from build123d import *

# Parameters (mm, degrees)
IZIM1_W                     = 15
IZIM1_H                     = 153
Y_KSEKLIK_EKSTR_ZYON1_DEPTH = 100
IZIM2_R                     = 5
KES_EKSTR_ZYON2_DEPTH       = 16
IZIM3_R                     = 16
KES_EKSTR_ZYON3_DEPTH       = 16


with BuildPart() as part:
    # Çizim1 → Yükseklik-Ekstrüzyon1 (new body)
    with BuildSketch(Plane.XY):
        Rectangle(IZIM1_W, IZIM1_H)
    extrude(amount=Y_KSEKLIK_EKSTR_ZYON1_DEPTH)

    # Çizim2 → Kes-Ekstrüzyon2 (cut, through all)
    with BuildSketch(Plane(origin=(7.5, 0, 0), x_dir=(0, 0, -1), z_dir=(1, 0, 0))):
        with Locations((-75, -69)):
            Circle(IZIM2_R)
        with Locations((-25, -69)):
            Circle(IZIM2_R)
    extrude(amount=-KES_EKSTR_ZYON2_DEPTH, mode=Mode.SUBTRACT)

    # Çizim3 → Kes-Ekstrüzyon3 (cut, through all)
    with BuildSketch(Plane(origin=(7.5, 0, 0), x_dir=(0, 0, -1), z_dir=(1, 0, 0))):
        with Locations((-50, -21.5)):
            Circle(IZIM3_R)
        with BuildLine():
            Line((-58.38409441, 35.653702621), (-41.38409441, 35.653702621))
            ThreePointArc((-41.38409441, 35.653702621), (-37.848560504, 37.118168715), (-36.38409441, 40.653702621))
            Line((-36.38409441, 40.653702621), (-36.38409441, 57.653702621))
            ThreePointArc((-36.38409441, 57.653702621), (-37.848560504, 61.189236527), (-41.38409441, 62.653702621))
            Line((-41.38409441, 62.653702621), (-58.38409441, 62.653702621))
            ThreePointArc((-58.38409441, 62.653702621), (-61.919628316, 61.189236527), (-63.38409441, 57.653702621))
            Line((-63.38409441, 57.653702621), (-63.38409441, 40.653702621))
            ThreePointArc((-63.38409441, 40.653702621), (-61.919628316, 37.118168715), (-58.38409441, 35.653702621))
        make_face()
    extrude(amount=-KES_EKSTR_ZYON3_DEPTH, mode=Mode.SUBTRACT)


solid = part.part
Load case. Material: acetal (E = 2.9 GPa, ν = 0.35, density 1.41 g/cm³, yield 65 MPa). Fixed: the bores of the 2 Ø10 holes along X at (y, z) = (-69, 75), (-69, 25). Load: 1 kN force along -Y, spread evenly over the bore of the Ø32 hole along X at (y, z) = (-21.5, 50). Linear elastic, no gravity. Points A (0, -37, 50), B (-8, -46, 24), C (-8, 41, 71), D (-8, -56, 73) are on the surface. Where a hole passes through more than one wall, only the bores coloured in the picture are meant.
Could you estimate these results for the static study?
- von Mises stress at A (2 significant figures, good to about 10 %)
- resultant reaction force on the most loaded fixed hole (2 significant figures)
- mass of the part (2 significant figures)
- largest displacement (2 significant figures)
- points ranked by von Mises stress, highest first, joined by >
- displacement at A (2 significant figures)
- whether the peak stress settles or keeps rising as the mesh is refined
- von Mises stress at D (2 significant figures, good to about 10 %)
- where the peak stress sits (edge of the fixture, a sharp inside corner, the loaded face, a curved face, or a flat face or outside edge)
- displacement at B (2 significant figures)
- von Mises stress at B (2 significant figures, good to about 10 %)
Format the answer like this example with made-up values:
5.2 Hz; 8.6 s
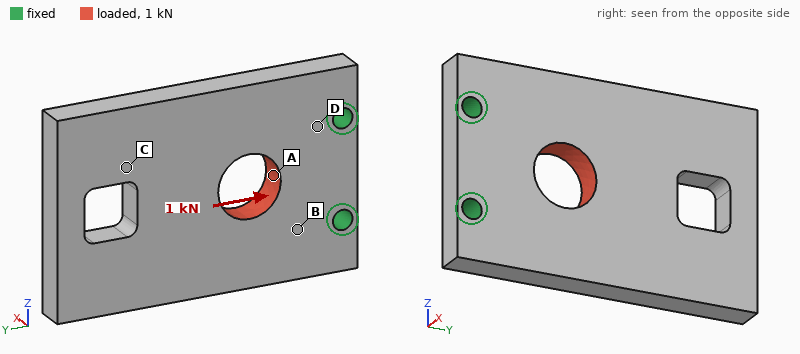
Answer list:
0.77 MPa; 500 N; 290 g; 25 µm; D > B > A > C; 11 µm; keeps rising; 1.4 MPa; edge of the fixture; 8.8 µm; 1.1 MPa
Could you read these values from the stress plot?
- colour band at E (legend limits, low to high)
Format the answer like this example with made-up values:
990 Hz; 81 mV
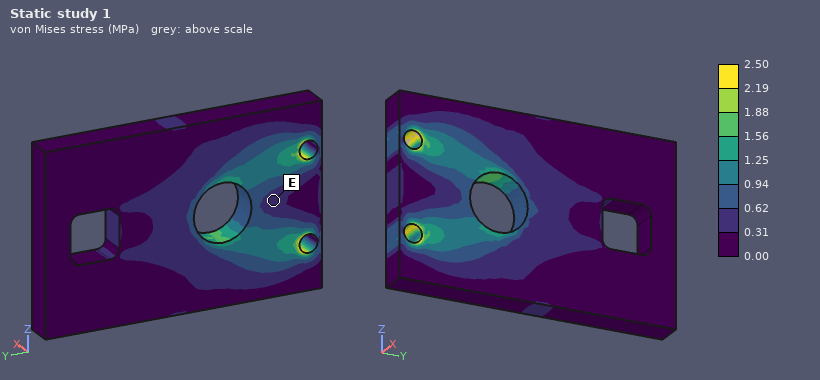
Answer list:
0.31 to 0.62 MPa
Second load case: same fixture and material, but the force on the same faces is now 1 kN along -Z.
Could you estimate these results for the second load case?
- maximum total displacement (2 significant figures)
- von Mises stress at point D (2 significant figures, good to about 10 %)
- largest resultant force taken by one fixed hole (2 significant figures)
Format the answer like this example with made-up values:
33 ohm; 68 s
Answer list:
0.18 mm; 2.1 MPa; 920 N
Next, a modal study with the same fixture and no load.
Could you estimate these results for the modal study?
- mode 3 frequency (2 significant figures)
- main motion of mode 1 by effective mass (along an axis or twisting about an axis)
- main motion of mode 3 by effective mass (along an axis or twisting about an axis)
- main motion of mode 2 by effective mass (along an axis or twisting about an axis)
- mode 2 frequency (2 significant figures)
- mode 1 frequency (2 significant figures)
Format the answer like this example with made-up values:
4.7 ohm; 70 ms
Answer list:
630 Hz; along X; along Z; twisting about Y; 450 Hz; 160 Hz
